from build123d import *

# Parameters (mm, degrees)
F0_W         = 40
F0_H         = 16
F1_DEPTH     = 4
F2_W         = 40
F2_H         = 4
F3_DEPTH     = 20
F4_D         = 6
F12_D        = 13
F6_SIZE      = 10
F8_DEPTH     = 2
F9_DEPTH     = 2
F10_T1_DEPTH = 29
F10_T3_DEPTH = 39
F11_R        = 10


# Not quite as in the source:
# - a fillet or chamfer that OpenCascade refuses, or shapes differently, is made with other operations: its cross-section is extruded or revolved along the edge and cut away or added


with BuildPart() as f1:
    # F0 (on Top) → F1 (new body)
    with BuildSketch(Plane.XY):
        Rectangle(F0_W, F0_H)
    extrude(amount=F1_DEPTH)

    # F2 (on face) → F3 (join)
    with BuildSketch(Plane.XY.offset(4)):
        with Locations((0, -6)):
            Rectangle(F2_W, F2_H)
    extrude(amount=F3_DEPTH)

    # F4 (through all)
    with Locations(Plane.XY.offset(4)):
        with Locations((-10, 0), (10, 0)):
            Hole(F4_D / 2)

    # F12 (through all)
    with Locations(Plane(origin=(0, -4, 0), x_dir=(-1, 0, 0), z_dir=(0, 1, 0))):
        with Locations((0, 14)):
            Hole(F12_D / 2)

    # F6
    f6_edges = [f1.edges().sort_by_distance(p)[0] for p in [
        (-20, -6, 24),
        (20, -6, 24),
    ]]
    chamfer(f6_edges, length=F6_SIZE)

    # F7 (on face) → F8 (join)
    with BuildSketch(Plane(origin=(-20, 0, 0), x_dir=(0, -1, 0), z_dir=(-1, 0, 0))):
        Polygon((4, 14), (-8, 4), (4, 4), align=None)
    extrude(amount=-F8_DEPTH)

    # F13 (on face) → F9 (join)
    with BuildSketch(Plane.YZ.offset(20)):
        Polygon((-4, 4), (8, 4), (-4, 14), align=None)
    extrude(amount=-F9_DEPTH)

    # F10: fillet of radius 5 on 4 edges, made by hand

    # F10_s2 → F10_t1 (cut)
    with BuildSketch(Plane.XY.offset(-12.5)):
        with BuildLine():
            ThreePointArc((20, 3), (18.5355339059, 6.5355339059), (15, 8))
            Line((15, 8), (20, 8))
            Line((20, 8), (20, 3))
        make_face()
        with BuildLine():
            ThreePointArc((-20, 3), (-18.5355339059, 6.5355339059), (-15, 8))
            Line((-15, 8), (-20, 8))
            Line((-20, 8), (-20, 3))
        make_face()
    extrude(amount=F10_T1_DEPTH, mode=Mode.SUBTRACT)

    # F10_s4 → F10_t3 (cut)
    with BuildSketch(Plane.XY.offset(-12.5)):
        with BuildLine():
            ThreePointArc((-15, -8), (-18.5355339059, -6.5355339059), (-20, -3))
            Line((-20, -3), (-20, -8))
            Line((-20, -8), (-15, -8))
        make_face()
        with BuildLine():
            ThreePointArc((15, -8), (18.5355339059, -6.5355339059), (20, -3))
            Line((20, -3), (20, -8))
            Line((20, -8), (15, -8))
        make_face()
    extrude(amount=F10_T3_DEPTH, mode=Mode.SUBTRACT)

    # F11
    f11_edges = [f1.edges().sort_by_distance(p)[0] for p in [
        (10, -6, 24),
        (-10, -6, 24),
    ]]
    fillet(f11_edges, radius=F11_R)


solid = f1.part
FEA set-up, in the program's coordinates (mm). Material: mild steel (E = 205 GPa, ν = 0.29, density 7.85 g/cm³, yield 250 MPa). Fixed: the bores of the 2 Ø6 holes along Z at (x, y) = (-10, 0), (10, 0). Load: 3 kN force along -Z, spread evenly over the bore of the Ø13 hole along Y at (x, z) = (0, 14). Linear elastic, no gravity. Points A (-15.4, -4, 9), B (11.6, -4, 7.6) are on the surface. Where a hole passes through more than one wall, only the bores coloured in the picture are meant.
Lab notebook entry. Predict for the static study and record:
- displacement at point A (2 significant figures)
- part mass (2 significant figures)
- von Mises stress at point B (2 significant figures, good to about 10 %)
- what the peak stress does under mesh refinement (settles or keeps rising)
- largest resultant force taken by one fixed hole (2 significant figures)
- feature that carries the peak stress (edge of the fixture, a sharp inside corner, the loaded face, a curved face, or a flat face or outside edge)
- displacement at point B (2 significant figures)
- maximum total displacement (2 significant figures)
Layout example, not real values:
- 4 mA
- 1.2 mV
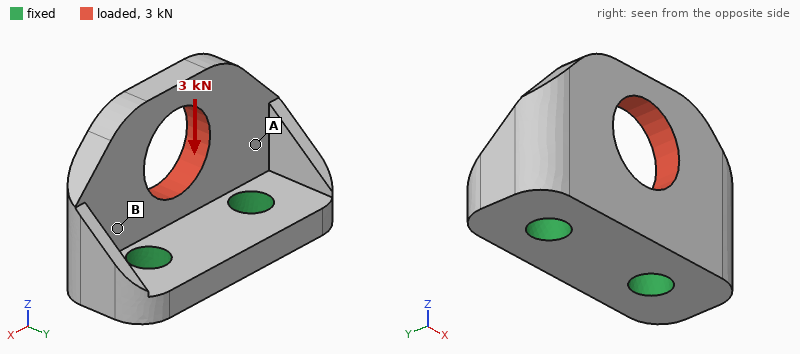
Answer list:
- 5.0 µm
- 36 g
- 36 MPa
- keeps rising
- 1.5 kN
- edge of the fixture
- 4.6 µm
- 19 µm
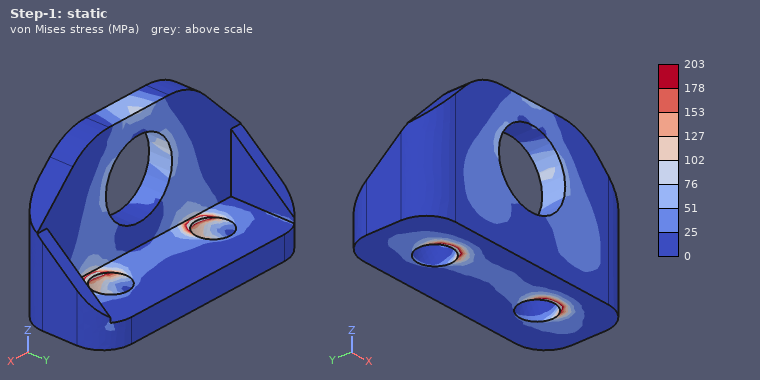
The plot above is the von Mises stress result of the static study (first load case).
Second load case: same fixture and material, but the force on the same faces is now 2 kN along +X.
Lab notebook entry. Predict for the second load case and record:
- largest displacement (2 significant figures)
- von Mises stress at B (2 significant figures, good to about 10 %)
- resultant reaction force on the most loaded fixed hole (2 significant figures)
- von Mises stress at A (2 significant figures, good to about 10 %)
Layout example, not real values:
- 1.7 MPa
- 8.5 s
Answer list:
- 14 µm
- 35 MPa
- 1.4 kN
- 28 MPa
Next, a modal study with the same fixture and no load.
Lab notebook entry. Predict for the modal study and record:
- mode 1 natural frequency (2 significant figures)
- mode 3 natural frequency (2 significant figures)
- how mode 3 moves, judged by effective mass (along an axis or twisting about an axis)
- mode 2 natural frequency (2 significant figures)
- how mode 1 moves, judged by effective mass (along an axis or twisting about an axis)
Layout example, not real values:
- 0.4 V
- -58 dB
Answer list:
- 7500 Hz
- 19 kHz
- along X
- 13 kHz
- along Y
